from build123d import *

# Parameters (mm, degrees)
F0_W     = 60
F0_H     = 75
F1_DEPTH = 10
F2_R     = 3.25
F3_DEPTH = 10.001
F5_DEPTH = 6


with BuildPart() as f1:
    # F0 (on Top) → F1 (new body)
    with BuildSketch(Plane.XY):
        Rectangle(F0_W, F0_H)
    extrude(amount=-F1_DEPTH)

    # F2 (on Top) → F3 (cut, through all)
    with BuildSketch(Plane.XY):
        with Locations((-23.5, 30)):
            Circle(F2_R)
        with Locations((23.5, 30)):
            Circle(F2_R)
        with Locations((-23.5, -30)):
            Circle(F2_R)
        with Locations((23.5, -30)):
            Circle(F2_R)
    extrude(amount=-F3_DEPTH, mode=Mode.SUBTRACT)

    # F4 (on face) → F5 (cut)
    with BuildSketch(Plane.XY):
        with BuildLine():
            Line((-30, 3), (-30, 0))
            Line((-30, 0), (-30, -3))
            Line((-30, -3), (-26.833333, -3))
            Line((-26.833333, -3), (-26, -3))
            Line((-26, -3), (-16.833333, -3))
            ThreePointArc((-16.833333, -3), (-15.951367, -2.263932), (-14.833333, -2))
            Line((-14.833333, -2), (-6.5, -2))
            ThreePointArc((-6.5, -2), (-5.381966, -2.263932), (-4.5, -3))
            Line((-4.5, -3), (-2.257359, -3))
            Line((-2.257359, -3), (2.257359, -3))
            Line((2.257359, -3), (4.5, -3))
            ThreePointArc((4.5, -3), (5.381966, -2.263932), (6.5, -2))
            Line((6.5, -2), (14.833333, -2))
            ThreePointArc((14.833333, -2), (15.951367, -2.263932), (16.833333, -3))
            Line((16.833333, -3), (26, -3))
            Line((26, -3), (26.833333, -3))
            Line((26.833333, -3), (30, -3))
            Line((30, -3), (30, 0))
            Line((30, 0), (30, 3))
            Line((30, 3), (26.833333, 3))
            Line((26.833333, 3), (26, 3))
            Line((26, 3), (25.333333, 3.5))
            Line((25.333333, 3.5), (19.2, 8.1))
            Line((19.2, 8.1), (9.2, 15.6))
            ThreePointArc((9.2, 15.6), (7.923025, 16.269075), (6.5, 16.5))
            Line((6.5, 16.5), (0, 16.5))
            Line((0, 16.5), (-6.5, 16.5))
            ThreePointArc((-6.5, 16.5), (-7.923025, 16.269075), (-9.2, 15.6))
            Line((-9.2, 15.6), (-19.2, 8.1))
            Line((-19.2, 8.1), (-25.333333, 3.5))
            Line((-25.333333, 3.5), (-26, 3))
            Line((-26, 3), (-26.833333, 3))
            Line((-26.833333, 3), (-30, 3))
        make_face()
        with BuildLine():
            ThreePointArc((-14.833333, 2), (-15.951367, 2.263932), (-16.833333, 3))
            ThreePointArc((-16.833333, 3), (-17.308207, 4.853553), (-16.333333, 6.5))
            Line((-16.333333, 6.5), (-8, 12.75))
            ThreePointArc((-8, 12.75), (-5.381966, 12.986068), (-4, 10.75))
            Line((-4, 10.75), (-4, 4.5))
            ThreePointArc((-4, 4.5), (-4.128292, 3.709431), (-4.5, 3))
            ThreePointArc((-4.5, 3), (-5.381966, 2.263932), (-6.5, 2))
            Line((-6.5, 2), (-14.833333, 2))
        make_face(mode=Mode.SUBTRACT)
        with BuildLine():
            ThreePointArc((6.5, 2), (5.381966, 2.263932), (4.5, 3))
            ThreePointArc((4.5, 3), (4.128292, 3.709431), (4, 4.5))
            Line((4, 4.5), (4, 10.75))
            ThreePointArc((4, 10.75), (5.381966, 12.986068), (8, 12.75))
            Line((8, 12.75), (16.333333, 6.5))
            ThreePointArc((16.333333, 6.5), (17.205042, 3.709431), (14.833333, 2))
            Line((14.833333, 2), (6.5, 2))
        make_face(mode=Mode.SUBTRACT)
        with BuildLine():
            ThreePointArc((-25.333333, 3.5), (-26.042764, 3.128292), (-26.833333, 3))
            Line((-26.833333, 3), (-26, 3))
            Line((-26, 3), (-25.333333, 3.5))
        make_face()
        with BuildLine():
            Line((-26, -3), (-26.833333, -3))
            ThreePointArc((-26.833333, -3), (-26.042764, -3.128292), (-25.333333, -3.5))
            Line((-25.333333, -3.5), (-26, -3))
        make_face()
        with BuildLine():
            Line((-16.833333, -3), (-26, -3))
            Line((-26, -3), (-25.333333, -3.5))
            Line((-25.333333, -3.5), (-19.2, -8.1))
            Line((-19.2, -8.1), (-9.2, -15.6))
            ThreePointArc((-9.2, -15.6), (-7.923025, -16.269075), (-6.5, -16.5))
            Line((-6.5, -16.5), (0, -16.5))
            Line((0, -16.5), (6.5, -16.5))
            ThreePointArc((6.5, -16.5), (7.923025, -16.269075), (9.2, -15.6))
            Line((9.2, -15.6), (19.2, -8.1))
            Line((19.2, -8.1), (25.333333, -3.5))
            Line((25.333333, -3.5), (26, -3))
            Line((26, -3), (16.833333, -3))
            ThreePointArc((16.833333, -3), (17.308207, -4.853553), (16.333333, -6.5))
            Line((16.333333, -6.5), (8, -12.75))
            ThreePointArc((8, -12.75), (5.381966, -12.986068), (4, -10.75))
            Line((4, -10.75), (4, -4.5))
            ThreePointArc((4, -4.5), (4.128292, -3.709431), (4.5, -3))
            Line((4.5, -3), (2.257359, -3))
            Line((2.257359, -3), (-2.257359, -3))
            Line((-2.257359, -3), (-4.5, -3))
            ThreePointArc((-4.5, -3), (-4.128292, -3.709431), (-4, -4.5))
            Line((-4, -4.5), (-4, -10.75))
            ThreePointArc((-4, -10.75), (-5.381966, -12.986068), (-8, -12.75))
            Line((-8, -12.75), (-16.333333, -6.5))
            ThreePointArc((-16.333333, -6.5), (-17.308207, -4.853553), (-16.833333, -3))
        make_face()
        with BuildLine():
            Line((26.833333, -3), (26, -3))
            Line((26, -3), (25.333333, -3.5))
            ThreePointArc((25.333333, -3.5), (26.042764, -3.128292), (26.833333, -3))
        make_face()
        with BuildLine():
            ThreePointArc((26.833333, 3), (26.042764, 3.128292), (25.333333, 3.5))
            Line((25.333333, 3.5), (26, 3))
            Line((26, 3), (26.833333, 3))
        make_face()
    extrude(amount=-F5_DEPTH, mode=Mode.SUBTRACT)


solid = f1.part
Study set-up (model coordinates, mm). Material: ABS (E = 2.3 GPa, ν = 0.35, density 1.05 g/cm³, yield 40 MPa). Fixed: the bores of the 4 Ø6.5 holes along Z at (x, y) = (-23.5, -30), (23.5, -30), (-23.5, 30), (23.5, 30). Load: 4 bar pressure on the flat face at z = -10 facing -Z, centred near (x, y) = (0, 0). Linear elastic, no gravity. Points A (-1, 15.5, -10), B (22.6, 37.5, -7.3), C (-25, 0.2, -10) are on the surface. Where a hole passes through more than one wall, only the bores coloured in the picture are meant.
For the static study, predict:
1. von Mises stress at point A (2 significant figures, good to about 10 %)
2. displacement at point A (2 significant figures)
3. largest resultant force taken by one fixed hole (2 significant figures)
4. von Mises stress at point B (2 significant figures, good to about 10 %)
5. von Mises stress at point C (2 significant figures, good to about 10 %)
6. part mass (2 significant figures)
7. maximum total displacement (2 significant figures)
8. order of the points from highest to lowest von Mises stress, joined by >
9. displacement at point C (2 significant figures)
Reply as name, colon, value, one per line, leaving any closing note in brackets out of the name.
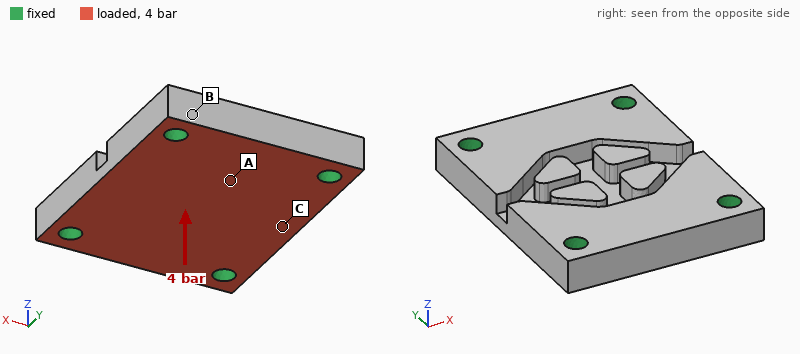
von Mises stress at point A: 3.3 MPa
displacement at point A: 0.15 mm
largest resultant force taken by one fixed hole: 510 N
von Mises stress at point B: 1.9 MPa
von Mises stress at point C: 7.3 MPa
part mass: 41 g
maximum total displacement: 0.26 mm
order of the points from highest to lowest von Mises stress, joined by >: C > A > B
displacement at point C: 0.16 mm
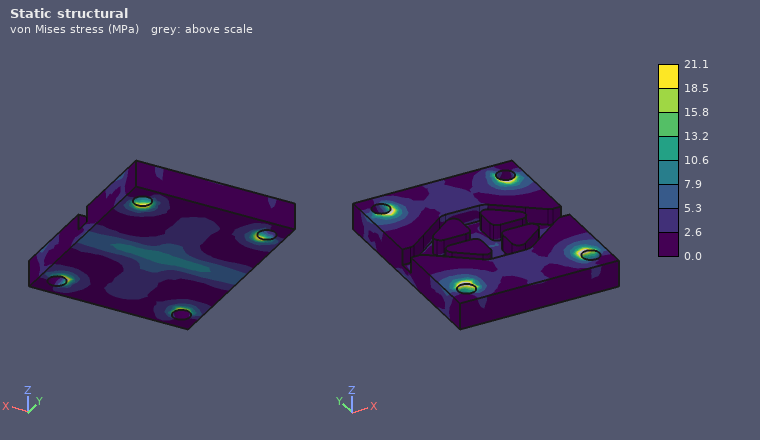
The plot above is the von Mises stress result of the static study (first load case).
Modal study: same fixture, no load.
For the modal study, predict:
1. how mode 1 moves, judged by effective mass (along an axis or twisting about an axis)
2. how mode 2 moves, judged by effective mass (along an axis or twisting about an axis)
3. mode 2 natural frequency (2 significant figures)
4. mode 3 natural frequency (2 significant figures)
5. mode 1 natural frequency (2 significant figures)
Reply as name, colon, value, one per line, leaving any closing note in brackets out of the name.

how mode 1 moves, judged by effective mass: along Z
how mode 2 moves, judged by effective mass: twisting about Y
mode 2 natural frequency: 4000 Hz
mode 3 natural frequency: 4700 Hz
mode 1 natural frequency: 2900 Hz
